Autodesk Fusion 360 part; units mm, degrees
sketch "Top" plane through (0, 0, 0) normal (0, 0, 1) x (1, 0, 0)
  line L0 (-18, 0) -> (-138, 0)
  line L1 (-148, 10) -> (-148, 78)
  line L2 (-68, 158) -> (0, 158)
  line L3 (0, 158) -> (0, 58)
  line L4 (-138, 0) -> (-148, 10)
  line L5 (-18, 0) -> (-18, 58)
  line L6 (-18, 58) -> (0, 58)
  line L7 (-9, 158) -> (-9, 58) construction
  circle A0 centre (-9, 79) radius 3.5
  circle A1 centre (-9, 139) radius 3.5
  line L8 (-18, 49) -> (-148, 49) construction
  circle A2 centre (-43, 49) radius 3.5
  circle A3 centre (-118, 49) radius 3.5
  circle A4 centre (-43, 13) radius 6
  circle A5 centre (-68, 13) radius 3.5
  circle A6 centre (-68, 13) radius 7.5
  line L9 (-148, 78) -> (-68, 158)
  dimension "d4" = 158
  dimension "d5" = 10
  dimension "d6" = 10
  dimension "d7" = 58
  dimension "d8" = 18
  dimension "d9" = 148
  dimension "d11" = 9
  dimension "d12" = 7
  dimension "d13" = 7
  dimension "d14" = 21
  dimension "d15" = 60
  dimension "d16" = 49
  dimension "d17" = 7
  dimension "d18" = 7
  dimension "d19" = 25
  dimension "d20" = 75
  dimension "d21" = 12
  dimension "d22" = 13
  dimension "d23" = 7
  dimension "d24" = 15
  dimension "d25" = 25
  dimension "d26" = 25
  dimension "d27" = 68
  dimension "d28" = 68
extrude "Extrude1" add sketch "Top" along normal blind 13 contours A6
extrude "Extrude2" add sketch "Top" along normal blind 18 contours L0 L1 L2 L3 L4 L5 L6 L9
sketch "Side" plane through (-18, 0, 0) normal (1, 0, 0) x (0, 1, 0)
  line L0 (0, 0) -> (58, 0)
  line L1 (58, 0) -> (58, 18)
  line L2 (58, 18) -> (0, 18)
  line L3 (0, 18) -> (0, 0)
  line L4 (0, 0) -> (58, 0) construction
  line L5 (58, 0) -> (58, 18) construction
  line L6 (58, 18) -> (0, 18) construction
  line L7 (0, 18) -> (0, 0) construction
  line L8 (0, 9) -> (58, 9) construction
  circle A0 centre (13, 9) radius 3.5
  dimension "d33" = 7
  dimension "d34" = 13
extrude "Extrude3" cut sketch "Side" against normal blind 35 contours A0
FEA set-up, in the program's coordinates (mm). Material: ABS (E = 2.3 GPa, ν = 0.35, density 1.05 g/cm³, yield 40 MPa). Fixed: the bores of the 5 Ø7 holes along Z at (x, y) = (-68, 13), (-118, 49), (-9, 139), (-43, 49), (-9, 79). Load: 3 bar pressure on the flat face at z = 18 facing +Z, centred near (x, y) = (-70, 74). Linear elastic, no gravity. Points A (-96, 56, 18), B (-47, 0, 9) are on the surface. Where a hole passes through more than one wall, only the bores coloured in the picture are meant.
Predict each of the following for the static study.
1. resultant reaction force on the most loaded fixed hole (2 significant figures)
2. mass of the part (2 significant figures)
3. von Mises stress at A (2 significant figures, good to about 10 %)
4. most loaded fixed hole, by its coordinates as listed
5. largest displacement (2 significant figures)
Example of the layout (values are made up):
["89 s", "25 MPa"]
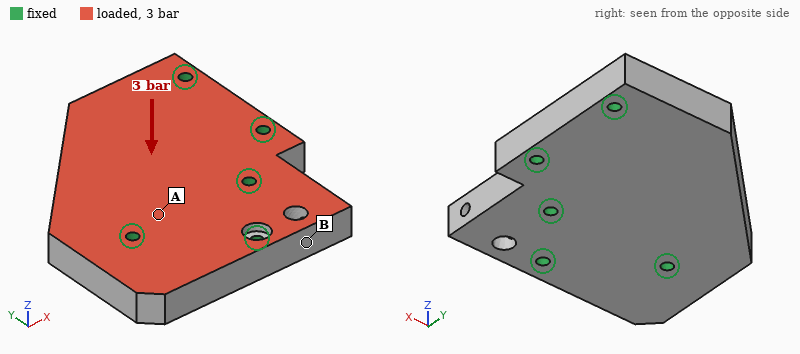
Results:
["2.1 kN", "350 g", "4.7 MPa", "(-118, 49)", "0.80 mm"]
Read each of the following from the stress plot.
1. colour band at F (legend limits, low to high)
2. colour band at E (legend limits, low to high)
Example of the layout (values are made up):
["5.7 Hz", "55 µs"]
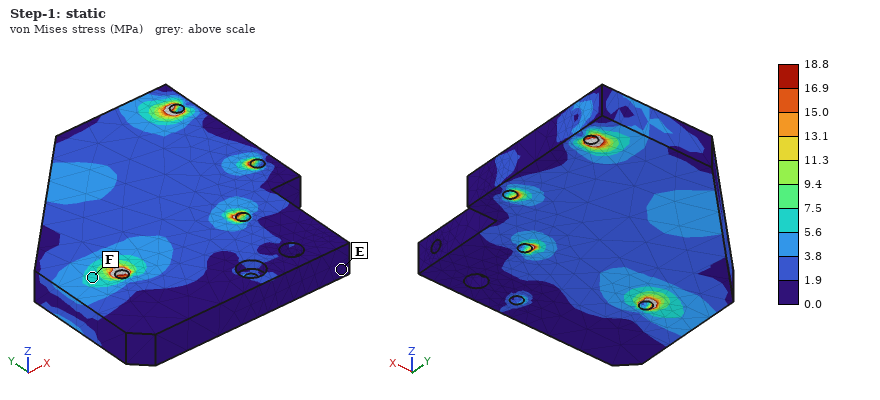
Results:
["5.6 to 7.5 MPa", "0.0 to 1.9 MPa"]
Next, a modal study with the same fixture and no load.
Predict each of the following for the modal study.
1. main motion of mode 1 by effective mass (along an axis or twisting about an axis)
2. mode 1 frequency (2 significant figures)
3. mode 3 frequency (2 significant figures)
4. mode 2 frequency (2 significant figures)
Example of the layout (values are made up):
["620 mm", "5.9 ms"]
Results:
["along Z", "920 Hz", "2100 Hz", "1800 Hz"]
